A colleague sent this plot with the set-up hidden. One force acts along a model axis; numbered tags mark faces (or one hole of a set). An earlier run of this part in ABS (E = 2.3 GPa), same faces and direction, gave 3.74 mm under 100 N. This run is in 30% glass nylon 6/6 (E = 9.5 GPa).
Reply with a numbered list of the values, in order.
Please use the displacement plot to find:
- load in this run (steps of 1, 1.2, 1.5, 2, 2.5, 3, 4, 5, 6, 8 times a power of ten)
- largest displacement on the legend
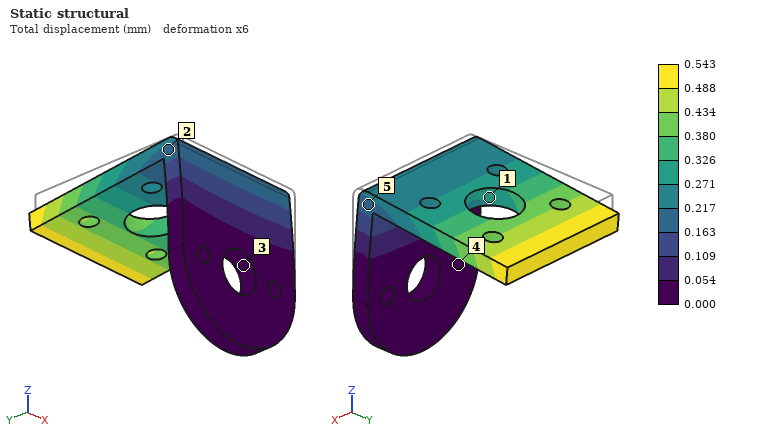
1. 60 N
2. 0.543 mm
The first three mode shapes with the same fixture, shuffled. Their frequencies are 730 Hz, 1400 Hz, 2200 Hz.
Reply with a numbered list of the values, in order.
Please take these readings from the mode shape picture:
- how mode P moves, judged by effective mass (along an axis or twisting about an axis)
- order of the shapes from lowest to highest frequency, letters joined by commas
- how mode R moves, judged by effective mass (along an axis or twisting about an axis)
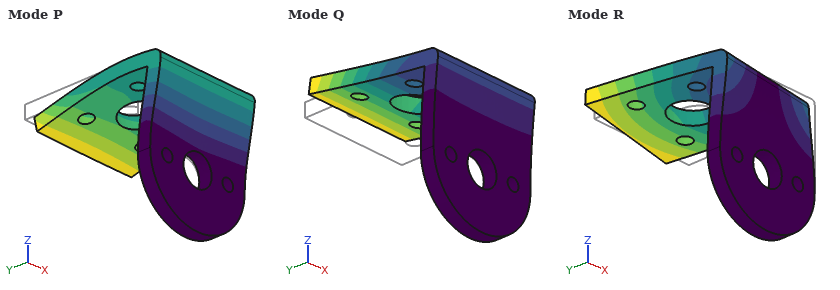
1. along Y
2. Q, R, P
3. along X
